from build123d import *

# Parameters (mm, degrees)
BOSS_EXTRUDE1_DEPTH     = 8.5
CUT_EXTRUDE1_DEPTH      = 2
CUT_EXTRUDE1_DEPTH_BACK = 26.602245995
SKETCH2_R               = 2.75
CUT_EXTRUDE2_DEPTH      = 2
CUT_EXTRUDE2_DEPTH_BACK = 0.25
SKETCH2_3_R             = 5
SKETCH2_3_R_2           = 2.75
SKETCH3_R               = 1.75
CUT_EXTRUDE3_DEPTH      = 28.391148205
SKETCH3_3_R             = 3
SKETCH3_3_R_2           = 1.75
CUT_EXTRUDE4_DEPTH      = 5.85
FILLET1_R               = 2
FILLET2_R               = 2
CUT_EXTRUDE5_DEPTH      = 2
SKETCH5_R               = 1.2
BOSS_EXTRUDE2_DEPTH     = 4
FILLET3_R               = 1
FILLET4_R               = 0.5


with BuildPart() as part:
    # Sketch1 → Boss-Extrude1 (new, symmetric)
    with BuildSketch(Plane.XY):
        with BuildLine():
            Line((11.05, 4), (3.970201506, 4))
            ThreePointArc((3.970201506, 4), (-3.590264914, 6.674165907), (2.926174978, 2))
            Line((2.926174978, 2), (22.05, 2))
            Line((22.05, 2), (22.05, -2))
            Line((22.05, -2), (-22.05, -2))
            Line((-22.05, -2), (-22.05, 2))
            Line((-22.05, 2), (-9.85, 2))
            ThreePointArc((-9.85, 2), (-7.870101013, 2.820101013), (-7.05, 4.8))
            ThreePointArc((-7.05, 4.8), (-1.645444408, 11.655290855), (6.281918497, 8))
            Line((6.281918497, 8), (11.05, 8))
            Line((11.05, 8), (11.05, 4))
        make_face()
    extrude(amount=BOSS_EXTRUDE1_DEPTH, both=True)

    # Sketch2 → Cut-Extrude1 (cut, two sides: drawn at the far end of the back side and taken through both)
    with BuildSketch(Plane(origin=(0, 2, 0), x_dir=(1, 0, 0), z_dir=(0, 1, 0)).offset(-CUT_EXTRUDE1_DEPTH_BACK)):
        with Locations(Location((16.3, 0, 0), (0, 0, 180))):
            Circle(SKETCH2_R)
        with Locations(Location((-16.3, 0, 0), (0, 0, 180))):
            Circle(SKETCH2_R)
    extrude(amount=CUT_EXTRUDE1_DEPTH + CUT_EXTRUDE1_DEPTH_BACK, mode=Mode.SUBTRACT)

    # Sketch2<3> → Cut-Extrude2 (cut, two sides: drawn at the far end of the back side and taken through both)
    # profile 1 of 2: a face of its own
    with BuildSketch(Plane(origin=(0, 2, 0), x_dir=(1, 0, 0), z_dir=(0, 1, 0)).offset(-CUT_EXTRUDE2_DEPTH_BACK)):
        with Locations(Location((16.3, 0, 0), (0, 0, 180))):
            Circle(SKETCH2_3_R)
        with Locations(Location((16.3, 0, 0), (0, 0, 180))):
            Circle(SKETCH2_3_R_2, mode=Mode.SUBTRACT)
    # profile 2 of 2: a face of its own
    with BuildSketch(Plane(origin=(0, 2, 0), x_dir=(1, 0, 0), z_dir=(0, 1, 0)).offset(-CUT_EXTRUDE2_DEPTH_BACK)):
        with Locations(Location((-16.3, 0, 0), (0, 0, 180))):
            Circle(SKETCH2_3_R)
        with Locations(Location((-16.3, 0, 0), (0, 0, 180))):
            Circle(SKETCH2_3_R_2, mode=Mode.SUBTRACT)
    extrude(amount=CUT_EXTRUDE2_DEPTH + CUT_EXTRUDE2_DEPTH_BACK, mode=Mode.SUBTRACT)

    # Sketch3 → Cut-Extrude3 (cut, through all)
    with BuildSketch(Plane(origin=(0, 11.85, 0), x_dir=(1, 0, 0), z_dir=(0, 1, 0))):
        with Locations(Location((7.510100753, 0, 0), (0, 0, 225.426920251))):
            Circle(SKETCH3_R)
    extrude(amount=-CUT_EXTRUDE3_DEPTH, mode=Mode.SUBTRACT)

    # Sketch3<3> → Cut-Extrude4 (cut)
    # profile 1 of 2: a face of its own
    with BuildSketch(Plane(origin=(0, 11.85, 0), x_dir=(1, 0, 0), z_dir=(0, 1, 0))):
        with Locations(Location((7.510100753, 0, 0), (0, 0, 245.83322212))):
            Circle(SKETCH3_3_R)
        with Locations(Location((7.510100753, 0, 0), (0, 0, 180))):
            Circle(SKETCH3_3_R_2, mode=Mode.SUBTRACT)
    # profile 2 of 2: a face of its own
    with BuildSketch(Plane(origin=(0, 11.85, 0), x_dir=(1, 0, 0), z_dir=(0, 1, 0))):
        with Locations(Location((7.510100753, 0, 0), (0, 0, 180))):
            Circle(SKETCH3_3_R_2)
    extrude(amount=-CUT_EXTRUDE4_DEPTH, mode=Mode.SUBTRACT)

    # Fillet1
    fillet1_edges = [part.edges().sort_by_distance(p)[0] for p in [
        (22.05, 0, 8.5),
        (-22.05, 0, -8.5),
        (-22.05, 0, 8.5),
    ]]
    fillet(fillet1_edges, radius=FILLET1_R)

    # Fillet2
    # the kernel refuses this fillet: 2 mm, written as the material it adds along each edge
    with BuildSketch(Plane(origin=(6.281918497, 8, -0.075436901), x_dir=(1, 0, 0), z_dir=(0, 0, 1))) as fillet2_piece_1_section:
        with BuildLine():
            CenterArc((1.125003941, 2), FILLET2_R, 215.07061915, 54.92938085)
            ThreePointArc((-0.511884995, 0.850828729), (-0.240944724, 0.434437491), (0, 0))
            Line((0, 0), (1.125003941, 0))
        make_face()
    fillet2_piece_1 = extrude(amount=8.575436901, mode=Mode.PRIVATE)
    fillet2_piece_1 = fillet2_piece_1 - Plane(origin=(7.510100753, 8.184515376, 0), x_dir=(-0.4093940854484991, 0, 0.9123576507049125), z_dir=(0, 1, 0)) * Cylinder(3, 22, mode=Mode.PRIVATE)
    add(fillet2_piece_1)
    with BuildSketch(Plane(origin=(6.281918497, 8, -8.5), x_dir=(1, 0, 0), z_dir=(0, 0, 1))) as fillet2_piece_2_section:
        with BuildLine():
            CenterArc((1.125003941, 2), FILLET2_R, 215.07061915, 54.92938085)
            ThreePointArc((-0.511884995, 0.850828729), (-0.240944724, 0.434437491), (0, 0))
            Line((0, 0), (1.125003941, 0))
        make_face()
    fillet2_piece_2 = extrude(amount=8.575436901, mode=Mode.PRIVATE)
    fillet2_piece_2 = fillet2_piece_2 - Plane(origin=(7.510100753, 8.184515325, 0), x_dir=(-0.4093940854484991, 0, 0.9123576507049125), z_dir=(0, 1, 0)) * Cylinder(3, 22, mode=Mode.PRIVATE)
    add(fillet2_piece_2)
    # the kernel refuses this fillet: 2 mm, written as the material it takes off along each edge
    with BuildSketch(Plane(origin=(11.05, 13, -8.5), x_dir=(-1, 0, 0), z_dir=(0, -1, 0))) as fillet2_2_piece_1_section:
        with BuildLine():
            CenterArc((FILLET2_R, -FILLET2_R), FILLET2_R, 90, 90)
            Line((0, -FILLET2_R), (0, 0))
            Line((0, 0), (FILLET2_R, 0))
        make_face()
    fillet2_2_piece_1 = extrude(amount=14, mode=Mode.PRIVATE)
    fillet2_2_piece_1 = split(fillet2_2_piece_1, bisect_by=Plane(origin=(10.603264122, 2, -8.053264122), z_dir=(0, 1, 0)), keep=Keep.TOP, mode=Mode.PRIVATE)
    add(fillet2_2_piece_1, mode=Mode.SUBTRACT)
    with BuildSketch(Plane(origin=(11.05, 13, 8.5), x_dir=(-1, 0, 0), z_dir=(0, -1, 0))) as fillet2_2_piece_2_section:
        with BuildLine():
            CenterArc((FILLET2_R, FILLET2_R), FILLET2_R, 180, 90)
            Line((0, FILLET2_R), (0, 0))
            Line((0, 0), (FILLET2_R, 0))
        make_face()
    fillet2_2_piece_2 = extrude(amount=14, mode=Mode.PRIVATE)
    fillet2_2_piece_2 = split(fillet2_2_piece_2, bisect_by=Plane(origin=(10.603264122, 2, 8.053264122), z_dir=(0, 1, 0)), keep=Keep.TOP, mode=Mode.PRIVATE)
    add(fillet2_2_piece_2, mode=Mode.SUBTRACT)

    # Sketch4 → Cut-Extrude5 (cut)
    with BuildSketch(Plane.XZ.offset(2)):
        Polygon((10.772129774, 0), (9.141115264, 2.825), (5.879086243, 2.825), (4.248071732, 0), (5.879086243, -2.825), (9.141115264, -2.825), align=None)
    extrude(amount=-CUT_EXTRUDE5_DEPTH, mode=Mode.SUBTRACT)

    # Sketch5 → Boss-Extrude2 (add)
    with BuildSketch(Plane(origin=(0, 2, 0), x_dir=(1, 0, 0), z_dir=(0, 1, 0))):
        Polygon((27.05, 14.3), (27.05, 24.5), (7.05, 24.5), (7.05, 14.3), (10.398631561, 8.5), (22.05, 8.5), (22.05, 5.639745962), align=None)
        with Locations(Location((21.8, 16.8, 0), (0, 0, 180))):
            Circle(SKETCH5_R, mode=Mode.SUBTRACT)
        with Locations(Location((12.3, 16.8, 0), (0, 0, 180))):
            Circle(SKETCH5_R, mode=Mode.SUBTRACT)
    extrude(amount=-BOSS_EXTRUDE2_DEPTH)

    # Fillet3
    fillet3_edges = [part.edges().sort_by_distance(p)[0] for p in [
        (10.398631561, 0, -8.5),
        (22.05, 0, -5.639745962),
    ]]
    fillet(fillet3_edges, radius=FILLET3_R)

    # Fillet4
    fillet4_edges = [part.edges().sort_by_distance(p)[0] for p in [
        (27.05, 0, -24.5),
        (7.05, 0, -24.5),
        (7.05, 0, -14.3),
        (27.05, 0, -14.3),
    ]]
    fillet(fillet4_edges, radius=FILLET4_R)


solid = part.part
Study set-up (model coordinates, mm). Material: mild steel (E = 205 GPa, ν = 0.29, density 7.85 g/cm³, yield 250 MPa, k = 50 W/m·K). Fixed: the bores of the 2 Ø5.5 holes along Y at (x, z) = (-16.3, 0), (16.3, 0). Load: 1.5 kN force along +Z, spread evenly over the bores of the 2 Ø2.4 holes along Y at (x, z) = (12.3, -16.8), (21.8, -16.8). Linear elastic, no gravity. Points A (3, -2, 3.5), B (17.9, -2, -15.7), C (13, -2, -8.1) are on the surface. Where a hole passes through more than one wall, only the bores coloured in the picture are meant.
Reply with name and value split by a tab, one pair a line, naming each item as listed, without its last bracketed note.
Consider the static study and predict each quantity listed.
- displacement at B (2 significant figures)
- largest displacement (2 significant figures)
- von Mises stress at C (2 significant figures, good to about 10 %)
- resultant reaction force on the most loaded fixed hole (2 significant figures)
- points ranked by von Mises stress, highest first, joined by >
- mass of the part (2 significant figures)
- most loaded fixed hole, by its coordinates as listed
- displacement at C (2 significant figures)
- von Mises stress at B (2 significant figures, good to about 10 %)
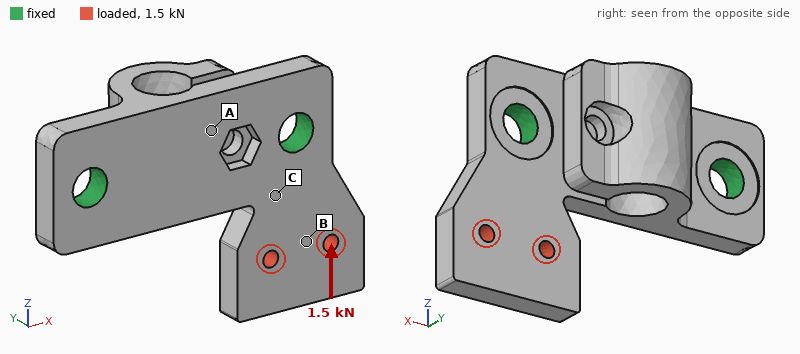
displacement at B	2.6 µm
largest displacement	4.5 µm
von Mises stress at C	26 MPa
resultant reaction force on the most loaded fixed hole	1.5 kN
points ranked by von Mises stress, highest first, joined by >	C > B > A
mass of the part	40 g
most loaded fixed hole, by its coordinates as listed	(16.3, 0)
displacement at C	0.80 µm
von Mises stress at B	18 MPa
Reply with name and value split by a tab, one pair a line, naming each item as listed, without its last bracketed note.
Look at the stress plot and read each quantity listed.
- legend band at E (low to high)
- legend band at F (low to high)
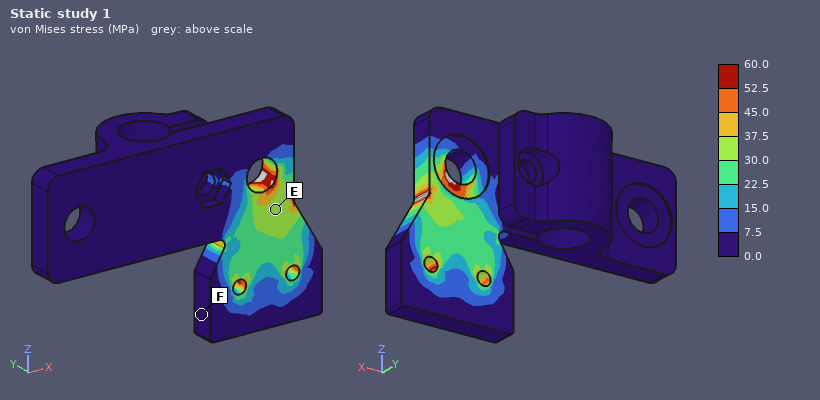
legend band at E	30.0 to 37.5 MPa
legend band at F	0.0 to 7.5 MPa
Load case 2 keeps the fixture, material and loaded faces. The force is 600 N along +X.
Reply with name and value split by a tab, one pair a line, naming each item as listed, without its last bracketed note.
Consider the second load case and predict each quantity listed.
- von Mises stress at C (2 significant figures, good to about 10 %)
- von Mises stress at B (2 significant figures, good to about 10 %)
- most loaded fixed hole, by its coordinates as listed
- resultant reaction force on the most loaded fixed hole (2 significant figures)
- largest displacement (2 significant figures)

von Mises stress at C	23 MPa
von Mises stress at B	19 MPa
most loaded fixed hole, by its coordinates as listed	(16.3, 0)
resultant reaction force on the most loaded fixed hole	420 N
largest displacement	12 µm
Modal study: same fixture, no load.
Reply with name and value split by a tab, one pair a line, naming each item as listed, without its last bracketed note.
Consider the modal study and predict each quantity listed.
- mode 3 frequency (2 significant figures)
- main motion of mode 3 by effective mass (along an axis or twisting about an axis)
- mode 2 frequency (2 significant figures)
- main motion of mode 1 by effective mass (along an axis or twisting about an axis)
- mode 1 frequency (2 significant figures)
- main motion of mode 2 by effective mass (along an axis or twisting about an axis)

mode 3 frequency	7900 Hz
main motion of mode 3 by effective mass	along Z
mode 2 frequency	5200 Hz
main motion of mode 1 by effective mass	along Y
mode 1 frequency	4700 Hz
main motion of mode 2 by effective mass	along Y
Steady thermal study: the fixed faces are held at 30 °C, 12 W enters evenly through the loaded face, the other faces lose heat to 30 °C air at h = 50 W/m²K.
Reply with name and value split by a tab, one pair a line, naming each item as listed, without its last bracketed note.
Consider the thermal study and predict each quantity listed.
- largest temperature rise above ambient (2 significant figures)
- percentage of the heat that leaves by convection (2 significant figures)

largest temperature rise above ambient	57 K
percentage of the heat that leaves by convection	19 %
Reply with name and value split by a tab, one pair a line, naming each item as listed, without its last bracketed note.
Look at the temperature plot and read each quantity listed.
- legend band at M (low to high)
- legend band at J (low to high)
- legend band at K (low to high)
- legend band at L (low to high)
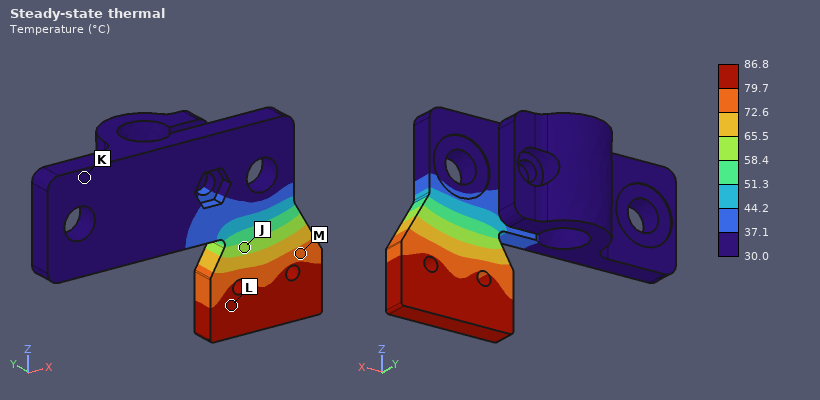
legend band at M	72.6 to 79.7 °C
legend band at J	58.4 to 65.5 °C
legend band at K	30.0 to 37.1 °C
legend band at L	79.7 to 86.8 °C
